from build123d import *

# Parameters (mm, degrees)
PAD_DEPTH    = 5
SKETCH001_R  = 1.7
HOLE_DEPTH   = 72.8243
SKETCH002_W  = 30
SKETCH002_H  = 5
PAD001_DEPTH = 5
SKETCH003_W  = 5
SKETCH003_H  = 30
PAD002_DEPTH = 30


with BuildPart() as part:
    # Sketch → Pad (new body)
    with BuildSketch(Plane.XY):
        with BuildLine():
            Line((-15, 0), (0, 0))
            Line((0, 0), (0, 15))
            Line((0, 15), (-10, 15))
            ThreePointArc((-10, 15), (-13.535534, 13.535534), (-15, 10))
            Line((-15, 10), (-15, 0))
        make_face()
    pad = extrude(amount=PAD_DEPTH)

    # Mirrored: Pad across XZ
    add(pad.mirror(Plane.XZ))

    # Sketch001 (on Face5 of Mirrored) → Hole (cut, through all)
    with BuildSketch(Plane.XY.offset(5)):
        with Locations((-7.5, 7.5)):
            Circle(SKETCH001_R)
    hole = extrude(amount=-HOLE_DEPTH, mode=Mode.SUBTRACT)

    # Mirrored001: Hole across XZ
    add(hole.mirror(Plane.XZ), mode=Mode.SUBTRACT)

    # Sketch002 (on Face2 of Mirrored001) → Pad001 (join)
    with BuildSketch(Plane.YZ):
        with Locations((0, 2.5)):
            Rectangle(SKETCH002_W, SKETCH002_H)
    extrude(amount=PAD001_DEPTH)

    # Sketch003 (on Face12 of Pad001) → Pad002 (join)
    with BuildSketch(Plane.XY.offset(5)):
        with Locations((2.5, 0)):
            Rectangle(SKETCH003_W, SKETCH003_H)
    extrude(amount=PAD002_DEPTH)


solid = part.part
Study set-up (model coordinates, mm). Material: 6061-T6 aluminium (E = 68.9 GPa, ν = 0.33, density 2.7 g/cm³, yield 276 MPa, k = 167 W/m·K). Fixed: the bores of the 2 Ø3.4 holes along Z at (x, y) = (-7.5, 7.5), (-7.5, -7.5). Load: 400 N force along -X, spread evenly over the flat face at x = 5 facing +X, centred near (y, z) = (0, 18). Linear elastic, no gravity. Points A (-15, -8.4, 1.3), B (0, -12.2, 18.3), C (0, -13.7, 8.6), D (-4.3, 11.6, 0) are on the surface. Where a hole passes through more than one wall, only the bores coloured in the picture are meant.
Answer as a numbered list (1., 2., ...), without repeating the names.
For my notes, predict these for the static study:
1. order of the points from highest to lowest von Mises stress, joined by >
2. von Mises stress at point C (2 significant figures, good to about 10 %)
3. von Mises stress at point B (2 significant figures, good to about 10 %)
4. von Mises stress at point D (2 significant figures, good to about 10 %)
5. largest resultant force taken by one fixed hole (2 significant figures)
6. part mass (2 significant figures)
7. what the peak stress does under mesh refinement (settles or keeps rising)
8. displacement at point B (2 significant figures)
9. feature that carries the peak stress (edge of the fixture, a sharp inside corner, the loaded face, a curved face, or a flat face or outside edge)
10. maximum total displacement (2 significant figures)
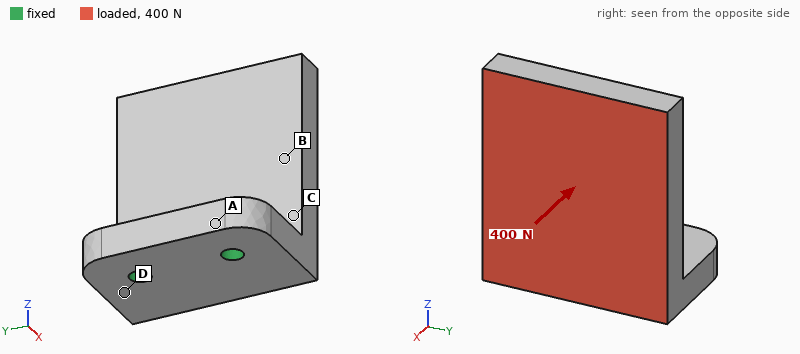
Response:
1. D > C > B > A
2. 28 MPa
3. 13 MPa
4. 37 MPa
5. 210 N
6. 20 g
7. keeps rising
8. 0.060 mm
9. edge of the fixture
10. 0.15 mm
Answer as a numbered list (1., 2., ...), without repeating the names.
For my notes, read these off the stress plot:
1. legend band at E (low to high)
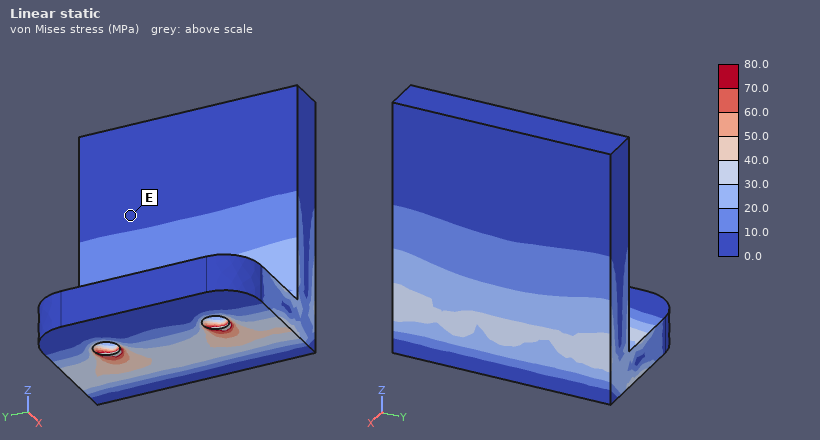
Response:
1. 0.0 to 10.0 MPa
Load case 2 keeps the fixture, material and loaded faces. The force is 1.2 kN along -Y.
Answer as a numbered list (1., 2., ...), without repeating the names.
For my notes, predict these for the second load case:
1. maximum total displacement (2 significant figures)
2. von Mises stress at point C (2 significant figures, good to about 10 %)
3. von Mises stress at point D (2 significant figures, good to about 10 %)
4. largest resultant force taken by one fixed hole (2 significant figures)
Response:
1. 78 µm
2. 41 MPa
3. 45 MPa
4. 1.4 kN
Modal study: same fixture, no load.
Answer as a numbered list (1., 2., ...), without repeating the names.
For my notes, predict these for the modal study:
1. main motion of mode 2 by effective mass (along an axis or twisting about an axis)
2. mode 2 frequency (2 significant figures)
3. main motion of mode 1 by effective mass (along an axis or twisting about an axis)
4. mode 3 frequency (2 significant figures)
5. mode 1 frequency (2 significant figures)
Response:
1. along Y
2. 5700 Hz
3. along X
4. 9000 Hz
5. 2700 Hz
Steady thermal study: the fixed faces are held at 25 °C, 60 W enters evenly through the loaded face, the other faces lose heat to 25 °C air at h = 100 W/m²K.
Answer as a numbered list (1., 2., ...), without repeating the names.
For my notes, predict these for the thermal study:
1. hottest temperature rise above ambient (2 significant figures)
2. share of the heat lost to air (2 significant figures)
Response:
1. 50 K
2. 11 %
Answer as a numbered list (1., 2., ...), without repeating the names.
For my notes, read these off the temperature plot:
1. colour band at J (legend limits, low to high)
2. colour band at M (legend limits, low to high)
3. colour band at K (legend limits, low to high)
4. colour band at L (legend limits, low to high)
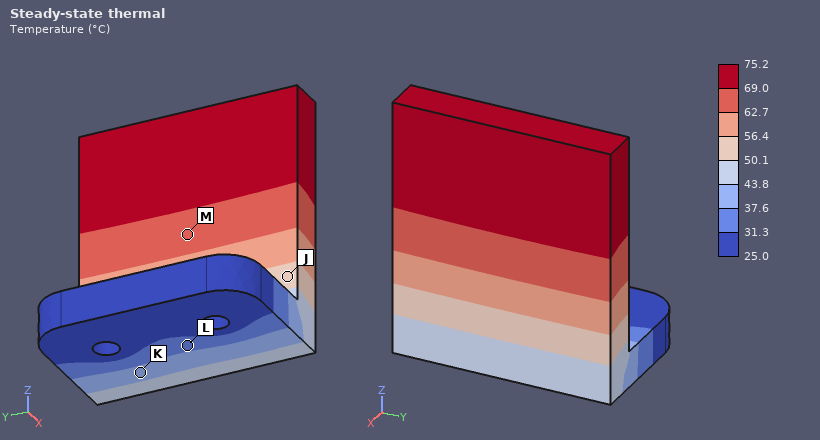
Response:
1. 50.1 to 56.4 °C
2. 62.7 to 69.0 °C
3. 37.6 to 43.8 °C
4. 31.3 to 37.6 °C
